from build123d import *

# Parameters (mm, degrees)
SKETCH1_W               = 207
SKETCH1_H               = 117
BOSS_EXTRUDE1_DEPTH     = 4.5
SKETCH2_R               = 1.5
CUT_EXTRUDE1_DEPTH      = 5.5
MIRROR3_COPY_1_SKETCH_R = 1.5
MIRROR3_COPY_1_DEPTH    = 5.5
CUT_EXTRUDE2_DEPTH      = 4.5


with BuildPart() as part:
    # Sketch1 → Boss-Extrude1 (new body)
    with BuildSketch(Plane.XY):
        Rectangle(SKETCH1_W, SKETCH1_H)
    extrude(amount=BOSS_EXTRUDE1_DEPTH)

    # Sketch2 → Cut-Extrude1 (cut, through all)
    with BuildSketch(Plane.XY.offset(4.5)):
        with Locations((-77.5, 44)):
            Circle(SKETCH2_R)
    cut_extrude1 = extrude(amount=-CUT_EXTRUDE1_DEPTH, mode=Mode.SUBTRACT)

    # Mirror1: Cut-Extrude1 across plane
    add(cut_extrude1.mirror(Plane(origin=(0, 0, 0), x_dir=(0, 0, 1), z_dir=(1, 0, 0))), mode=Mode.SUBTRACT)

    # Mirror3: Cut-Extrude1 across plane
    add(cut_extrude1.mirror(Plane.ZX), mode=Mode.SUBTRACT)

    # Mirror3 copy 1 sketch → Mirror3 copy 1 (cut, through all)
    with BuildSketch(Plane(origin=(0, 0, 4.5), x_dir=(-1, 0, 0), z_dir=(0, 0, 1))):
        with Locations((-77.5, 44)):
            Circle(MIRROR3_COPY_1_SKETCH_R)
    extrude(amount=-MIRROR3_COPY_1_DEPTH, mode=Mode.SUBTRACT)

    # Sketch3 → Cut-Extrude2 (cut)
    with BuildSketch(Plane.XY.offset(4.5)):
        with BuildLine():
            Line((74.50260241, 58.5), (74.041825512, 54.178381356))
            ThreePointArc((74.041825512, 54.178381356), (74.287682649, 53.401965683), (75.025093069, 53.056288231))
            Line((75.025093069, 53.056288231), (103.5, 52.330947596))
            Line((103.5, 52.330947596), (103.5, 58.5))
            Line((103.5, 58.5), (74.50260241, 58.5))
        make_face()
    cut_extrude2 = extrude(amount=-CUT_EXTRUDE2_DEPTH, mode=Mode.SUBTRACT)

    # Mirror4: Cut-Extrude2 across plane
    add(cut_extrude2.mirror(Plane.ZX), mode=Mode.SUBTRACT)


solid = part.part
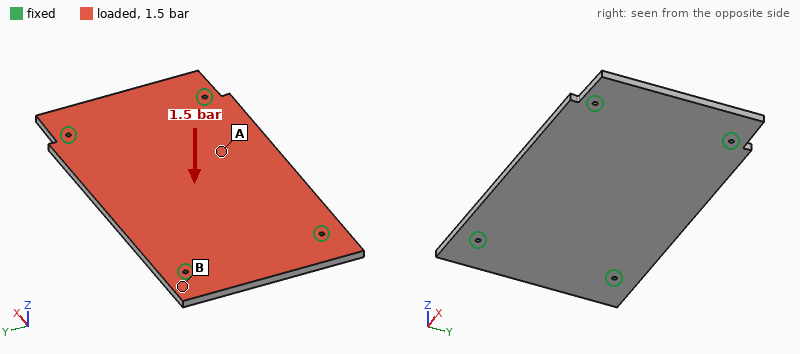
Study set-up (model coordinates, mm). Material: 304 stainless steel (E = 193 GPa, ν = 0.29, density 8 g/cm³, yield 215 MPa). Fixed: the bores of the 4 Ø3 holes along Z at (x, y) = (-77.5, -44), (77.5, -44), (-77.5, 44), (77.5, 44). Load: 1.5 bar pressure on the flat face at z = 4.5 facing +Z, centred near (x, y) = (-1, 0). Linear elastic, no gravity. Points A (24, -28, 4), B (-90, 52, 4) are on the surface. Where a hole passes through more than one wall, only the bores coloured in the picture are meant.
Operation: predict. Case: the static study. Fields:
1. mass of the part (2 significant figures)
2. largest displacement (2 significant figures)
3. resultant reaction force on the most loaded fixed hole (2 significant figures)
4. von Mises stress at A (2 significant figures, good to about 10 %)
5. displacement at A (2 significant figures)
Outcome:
860 g
0.23 mm
910 N
39 MPa
0.20 mm
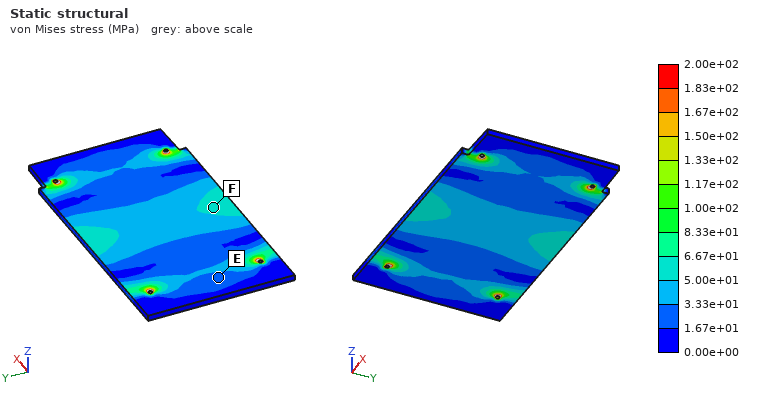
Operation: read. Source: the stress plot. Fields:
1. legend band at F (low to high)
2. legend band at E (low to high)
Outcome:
5.00e+01 to 6.67e+01 MPa
1.67e+01 to 3.33e+01 MPa
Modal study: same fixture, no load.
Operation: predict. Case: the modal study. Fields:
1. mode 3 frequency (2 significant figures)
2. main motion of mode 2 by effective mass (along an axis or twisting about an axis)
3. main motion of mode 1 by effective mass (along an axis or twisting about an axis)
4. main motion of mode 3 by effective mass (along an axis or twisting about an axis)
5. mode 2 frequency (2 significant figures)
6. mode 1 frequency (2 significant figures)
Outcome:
2000 Hz
twisting about X
along Z
twisting about Y
1200 Hz
750 Hz
